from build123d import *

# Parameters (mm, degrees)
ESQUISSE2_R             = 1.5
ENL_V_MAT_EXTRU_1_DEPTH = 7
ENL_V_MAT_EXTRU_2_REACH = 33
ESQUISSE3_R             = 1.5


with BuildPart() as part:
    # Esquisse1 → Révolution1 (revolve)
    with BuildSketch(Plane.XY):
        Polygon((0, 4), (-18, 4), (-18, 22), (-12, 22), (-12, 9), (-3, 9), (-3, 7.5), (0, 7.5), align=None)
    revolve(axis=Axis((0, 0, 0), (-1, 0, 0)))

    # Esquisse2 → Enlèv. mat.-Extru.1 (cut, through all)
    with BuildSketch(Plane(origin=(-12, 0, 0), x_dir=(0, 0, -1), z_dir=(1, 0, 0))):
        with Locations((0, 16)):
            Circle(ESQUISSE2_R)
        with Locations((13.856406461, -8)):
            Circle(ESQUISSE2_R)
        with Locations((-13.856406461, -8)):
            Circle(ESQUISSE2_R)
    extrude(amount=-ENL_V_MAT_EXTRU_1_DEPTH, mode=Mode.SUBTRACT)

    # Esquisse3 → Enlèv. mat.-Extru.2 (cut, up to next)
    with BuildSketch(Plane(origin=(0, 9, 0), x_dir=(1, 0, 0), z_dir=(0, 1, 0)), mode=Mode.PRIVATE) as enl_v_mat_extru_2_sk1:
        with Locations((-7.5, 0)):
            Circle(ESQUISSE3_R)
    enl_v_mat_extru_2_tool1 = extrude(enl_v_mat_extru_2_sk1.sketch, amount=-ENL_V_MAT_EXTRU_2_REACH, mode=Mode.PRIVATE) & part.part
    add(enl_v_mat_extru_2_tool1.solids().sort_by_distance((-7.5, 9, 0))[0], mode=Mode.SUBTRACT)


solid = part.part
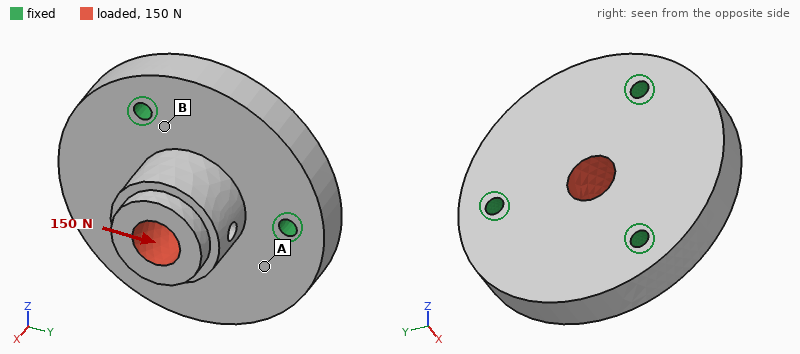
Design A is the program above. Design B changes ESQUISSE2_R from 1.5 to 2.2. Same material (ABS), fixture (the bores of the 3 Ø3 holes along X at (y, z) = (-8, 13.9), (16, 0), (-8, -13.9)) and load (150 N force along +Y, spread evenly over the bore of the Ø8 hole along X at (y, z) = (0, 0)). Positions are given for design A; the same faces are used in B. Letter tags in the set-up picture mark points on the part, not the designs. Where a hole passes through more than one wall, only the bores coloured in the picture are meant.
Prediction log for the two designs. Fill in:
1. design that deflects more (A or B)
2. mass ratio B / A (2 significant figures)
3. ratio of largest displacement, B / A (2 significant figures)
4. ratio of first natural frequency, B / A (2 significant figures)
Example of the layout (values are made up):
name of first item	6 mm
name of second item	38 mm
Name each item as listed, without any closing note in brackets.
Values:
design that deflects more	A
mass ratio B / A	0.99
ratio of largest displacement, B / A	0.91
ratio of first natural frequency, B / A	1.1
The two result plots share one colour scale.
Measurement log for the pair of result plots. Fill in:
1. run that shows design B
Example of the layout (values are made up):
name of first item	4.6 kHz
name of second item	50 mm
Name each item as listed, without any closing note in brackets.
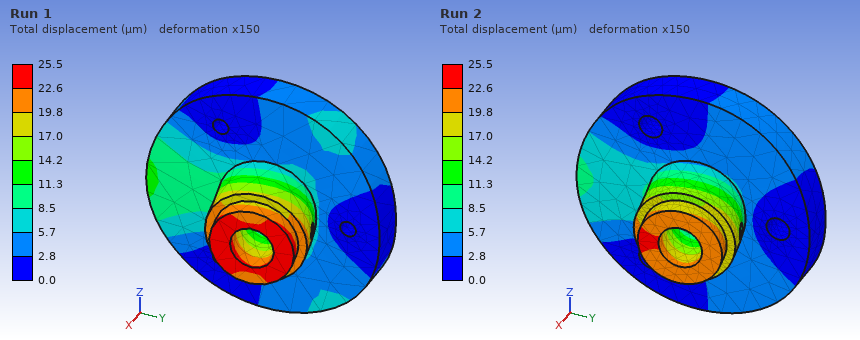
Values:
run that shows design B	Run 2
